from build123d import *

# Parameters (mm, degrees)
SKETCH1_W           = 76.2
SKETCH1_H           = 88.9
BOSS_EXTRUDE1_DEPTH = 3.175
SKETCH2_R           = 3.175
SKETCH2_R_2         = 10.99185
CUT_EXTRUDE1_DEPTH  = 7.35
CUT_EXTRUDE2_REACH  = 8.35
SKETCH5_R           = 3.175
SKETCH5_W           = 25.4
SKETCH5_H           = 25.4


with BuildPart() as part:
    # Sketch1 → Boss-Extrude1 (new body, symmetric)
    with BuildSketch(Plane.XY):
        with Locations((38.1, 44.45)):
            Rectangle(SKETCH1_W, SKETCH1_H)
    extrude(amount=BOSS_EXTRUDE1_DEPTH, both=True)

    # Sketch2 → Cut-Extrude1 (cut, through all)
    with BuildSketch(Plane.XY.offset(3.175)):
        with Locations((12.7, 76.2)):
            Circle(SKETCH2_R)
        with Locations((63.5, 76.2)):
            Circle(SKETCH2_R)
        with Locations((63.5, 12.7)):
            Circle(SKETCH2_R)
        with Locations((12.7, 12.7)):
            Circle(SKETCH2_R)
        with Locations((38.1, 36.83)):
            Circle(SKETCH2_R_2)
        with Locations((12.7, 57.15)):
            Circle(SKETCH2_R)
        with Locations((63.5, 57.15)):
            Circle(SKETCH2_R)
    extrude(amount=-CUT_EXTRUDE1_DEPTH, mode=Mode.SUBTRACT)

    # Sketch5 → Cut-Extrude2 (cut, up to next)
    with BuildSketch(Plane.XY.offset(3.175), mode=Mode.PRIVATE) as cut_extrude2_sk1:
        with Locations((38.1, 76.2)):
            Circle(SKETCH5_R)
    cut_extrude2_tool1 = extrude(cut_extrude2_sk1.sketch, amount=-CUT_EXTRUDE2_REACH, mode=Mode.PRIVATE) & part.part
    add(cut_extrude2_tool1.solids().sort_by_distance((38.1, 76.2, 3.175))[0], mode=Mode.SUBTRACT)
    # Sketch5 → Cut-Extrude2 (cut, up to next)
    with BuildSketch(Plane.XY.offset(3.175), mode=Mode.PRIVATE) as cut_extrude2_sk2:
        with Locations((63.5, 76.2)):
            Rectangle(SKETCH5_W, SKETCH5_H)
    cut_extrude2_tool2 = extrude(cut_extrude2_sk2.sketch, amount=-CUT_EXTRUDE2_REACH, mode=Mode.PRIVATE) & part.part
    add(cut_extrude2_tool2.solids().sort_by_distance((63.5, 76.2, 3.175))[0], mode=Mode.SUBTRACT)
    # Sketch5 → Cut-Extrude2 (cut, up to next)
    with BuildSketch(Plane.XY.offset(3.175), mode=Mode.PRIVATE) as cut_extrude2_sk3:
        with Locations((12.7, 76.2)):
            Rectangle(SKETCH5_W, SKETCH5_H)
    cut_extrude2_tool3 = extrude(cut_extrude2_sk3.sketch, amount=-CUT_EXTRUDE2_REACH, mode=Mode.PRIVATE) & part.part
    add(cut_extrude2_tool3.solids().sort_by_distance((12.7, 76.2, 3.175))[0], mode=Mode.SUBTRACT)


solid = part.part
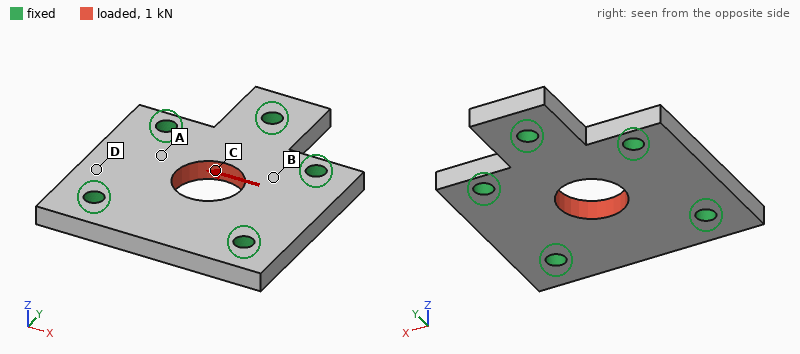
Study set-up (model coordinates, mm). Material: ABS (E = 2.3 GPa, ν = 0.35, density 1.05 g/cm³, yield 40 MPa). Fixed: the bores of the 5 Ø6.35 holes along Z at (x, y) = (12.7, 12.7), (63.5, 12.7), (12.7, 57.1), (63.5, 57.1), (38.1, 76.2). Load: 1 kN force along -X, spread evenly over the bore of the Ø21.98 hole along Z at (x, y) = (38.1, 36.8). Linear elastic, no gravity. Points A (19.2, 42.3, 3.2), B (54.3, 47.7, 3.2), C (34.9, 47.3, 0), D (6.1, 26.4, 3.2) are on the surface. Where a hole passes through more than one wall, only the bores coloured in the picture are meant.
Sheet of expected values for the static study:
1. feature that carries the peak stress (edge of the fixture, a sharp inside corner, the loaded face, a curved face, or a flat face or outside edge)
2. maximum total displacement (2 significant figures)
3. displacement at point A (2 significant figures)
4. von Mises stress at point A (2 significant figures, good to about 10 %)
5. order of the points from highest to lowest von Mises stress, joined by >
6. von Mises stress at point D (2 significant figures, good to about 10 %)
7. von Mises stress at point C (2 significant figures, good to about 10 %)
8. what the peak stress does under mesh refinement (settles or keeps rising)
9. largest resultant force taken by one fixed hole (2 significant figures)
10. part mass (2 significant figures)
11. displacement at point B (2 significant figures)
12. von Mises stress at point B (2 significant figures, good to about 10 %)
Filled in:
edge of the fixture
31 µm
22 µm
1.8 MPa
C > B > A > D
1.0 MPa
3.9 MPa
keeps rising
260 N
33 g
16 µm
2.4 MPa
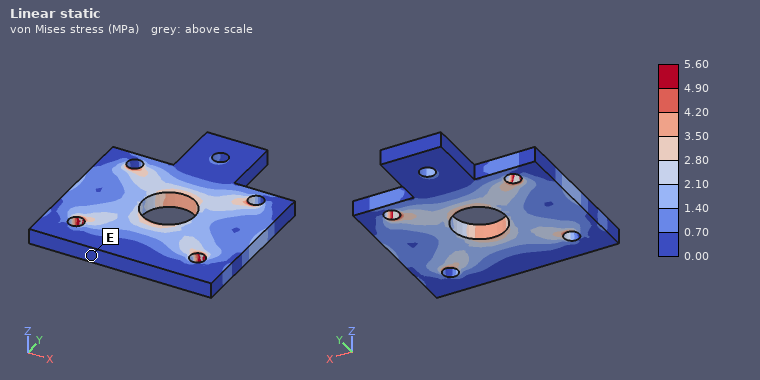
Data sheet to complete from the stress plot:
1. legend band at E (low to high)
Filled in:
0.00 to 0.70 MPa
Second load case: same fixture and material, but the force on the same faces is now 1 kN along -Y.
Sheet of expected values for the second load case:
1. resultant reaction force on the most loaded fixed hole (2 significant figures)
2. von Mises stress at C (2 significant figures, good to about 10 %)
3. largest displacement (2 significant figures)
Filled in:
240 N
2.2 MPa
37 µm
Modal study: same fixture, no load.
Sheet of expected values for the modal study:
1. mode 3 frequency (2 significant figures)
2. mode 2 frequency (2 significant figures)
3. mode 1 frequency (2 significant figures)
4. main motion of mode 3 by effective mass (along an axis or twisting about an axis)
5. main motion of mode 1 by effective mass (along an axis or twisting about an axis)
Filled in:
4500 Hz
3900 Hz
3300 Hz
twisting about Y
along Z
